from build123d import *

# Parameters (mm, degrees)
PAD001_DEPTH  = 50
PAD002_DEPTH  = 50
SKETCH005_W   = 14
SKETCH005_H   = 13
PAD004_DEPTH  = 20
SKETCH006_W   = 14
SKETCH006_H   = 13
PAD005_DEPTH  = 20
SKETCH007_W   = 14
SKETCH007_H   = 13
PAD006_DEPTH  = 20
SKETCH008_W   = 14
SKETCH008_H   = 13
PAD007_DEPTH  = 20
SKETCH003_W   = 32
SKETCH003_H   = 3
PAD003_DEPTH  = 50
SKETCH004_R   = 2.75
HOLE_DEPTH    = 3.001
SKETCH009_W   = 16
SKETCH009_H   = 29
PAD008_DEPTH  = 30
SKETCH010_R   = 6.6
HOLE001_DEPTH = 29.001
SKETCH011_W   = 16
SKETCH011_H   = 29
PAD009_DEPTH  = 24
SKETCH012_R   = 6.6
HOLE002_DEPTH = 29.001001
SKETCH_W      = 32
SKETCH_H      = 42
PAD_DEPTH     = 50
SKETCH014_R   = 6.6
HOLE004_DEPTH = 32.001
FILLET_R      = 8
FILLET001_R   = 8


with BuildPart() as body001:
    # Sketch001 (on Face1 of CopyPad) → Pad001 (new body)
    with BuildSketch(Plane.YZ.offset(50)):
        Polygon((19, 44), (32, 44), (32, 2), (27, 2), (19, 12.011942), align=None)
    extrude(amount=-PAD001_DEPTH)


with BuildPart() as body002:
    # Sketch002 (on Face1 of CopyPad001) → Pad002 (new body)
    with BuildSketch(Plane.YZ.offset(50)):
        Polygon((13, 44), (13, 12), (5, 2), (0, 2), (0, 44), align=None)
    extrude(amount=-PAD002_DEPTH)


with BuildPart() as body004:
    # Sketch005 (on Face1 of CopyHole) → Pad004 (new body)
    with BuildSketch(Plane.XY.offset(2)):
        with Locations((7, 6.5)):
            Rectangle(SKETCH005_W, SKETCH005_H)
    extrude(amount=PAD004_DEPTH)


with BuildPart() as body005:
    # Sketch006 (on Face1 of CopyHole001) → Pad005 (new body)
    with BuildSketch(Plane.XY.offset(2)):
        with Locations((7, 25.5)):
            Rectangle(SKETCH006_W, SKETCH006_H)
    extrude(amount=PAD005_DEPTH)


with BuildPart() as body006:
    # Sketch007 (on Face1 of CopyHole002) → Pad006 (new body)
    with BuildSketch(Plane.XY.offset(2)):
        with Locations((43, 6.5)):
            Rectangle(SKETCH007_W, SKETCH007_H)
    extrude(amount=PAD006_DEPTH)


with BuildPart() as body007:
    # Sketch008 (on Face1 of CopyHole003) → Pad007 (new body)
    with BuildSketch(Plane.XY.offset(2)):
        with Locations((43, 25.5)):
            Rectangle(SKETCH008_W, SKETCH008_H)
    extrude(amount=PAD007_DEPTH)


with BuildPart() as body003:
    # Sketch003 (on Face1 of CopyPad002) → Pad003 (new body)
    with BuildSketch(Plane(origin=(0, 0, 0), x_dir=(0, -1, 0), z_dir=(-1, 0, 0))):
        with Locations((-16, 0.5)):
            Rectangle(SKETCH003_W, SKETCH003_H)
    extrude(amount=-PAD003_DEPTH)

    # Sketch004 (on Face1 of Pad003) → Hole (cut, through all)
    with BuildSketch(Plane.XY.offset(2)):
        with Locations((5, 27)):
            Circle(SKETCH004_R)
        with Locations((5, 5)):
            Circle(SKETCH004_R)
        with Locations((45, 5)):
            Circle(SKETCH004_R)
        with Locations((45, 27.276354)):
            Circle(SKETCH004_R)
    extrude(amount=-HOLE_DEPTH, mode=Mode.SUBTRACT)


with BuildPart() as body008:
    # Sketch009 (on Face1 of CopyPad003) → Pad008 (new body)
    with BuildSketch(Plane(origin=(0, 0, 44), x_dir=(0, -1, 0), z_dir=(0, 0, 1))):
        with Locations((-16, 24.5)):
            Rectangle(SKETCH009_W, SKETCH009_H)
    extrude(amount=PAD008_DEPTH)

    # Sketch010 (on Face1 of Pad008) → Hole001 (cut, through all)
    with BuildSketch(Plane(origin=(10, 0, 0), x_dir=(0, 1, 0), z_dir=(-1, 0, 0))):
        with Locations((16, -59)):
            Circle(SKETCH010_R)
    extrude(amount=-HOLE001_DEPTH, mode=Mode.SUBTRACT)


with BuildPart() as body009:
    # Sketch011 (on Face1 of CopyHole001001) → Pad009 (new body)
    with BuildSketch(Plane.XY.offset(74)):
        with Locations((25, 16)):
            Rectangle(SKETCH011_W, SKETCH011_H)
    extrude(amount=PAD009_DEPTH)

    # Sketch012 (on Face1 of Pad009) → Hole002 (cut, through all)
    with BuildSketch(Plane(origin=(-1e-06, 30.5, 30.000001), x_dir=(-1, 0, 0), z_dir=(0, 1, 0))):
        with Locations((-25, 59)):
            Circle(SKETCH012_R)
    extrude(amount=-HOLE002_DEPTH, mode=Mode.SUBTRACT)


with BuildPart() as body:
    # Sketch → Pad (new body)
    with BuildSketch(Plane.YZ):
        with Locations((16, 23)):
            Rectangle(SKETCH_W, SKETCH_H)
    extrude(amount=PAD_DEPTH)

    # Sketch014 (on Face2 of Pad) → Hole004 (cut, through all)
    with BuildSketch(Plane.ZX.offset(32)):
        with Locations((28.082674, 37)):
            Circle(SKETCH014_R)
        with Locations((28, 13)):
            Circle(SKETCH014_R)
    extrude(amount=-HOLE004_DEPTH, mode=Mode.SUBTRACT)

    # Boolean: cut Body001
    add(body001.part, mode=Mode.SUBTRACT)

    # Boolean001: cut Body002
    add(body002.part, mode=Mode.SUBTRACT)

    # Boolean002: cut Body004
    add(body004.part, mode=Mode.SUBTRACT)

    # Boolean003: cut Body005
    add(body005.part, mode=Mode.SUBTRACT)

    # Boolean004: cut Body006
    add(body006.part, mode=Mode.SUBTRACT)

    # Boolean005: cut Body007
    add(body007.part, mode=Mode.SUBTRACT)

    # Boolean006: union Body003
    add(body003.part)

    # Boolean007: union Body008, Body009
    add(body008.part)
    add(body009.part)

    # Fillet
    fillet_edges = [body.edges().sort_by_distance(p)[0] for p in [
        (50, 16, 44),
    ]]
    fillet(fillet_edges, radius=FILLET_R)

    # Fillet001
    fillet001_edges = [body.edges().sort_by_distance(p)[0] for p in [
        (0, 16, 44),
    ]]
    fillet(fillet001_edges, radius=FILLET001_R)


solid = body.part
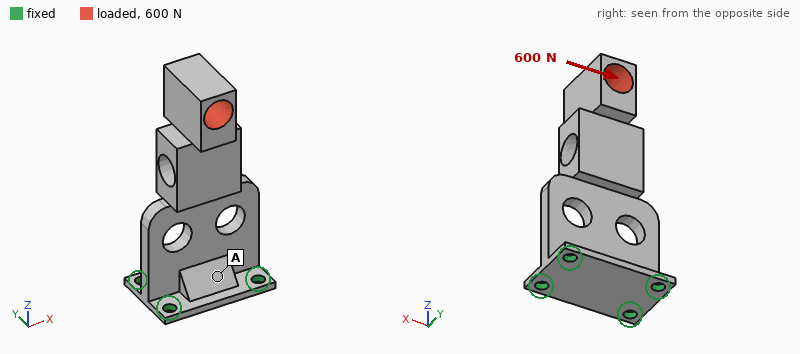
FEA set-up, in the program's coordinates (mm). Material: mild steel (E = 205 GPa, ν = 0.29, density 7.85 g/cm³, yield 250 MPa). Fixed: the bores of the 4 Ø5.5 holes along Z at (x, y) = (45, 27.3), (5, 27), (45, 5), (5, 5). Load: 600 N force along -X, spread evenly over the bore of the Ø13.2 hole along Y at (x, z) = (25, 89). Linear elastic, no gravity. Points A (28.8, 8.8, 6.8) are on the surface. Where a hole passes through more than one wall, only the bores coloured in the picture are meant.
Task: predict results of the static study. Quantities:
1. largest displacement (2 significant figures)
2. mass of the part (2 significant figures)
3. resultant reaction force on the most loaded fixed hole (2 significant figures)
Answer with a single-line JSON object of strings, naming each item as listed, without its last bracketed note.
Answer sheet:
{"largest displacement": "67 µm", "mass of the part": "270 g", "resultant reaction force on the most loaded fixed hole": "750 N"}
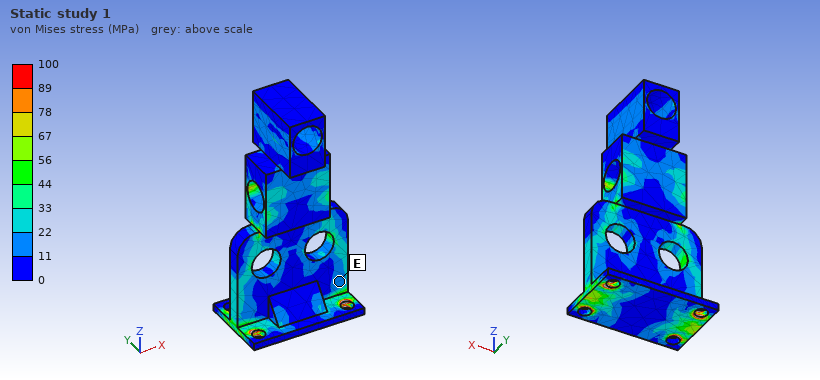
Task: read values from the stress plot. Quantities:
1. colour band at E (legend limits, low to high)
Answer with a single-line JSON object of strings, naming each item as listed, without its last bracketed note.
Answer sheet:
{"colour band at E": "11 to 22 MPa"}
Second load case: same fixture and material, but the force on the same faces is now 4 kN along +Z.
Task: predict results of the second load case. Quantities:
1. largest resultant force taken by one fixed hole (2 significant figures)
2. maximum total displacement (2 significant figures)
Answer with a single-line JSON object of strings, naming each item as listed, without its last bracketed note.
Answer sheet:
{"largest resultant force taken by one fixed hole": "1.1 kN", "maximum total displacement": "22 µm"}
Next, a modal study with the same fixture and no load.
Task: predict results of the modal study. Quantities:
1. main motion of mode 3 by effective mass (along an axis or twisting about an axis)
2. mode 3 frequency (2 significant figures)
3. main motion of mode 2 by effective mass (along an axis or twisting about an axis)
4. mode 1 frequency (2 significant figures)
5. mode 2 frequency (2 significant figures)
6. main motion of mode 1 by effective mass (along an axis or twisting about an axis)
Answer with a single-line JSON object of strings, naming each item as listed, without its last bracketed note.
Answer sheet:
{"main motion of mode 3 by effective mass": "twisting about Z", "mode 3 frequency": "3200 Hz", "main motion of mode 2 by effective mass": "along X", "mode 1 frequency": "480 Hz", "mode 2 frequency": "1900 Hz", "main motion of mode 1 by effective mass": "along Y"}
